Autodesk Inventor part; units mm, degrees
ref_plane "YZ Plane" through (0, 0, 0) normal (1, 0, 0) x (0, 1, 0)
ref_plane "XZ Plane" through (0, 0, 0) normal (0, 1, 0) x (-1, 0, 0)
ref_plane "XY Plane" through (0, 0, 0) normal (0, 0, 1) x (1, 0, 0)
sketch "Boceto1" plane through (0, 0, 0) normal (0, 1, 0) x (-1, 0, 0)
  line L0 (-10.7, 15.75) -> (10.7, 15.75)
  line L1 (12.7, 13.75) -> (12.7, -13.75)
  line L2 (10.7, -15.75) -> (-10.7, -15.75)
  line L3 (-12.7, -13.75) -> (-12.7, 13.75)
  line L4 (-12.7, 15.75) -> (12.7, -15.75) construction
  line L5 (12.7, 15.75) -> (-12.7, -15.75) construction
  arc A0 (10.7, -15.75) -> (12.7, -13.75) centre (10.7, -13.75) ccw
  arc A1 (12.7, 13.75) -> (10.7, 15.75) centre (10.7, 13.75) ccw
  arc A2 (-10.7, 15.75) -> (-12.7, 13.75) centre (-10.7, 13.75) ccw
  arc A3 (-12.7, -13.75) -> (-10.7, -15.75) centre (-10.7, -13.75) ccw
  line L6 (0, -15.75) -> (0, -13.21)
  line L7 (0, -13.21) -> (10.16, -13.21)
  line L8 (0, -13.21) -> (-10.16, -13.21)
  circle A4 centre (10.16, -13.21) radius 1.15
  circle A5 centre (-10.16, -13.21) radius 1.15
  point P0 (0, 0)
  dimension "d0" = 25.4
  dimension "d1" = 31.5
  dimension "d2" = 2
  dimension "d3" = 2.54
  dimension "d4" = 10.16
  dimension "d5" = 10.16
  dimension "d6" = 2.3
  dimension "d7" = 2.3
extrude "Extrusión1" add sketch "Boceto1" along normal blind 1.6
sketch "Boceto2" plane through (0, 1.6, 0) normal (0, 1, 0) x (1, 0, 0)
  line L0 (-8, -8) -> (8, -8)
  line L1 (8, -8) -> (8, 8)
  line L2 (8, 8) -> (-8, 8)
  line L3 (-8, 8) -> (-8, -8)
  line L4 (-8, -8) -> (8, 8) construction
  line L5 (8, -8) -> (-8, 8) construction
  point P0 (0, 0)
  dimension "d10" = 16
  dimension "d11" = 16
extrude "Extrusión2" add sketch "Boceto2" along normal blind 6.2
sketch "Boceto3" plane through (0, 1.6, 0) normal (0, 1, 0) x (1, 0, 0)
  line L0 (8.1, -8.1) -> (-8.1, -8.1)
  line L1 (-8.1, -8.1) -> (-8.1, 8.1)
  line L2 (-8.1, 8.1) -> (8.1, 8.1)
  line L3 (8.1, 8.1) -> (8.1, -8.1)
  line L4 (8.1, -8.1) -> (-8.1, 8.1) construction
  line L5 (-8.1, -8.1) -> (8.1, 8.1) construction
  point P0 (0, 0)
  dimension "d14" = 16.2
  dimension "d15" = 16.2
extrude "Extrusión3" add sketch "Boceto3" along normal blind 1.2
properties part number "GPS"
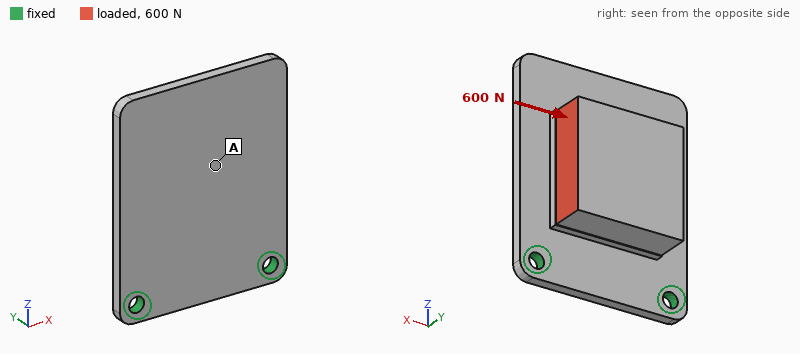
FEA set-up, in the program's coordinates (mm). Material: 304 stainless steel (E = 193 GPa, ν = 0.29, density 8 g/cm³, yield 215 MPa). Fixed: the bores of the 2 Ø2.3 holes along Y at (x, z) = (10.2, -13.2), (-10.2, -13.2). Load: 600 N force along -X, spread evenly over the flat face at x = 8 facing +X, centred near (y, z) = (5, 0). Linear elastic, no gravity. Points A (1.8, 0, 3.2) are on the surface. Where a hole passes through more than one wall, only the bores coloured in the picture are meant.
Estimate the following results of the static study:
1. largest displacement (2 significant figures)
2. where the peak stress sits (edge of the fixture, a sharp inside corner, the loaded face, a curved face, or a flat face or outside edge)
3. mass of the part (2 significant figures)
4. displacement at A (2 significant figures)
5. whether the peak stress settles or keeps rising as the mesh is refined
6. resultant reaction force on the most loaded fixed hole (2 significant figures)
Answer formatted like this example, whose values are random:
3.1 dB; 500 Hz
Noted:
13 µm; edge of the fixture; 23 g; 2.8 µm; keeps rising; 500 N
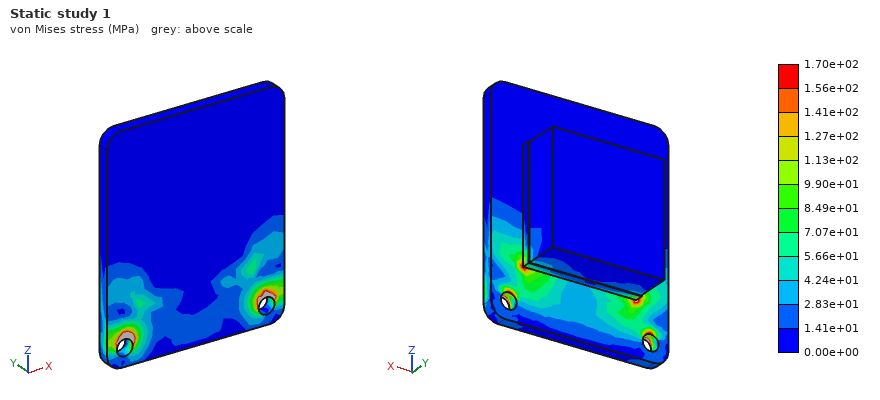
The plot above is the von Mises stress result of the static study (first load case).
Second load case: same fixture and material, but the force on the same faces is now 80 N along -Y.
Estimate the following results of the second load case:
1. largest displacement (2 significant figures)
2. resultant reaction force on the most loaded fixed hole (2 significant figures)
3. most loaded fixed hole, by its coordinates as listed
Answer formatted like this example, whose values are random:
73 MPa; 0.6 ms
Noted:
94 µm; 75 N; (10.2, -13.2)
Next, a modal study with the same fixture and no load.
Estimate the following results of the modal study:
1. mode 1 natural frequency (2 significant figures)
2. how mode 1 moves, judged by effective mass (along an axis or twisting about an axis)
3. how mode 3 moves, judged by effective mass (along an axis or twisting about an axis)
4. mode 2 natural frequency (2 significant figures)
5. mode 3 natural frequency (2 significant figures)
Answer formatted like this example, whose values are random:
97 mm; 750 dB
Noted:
1300 Hz; along Y; along Y; 8200 Hz; 12 kHz
